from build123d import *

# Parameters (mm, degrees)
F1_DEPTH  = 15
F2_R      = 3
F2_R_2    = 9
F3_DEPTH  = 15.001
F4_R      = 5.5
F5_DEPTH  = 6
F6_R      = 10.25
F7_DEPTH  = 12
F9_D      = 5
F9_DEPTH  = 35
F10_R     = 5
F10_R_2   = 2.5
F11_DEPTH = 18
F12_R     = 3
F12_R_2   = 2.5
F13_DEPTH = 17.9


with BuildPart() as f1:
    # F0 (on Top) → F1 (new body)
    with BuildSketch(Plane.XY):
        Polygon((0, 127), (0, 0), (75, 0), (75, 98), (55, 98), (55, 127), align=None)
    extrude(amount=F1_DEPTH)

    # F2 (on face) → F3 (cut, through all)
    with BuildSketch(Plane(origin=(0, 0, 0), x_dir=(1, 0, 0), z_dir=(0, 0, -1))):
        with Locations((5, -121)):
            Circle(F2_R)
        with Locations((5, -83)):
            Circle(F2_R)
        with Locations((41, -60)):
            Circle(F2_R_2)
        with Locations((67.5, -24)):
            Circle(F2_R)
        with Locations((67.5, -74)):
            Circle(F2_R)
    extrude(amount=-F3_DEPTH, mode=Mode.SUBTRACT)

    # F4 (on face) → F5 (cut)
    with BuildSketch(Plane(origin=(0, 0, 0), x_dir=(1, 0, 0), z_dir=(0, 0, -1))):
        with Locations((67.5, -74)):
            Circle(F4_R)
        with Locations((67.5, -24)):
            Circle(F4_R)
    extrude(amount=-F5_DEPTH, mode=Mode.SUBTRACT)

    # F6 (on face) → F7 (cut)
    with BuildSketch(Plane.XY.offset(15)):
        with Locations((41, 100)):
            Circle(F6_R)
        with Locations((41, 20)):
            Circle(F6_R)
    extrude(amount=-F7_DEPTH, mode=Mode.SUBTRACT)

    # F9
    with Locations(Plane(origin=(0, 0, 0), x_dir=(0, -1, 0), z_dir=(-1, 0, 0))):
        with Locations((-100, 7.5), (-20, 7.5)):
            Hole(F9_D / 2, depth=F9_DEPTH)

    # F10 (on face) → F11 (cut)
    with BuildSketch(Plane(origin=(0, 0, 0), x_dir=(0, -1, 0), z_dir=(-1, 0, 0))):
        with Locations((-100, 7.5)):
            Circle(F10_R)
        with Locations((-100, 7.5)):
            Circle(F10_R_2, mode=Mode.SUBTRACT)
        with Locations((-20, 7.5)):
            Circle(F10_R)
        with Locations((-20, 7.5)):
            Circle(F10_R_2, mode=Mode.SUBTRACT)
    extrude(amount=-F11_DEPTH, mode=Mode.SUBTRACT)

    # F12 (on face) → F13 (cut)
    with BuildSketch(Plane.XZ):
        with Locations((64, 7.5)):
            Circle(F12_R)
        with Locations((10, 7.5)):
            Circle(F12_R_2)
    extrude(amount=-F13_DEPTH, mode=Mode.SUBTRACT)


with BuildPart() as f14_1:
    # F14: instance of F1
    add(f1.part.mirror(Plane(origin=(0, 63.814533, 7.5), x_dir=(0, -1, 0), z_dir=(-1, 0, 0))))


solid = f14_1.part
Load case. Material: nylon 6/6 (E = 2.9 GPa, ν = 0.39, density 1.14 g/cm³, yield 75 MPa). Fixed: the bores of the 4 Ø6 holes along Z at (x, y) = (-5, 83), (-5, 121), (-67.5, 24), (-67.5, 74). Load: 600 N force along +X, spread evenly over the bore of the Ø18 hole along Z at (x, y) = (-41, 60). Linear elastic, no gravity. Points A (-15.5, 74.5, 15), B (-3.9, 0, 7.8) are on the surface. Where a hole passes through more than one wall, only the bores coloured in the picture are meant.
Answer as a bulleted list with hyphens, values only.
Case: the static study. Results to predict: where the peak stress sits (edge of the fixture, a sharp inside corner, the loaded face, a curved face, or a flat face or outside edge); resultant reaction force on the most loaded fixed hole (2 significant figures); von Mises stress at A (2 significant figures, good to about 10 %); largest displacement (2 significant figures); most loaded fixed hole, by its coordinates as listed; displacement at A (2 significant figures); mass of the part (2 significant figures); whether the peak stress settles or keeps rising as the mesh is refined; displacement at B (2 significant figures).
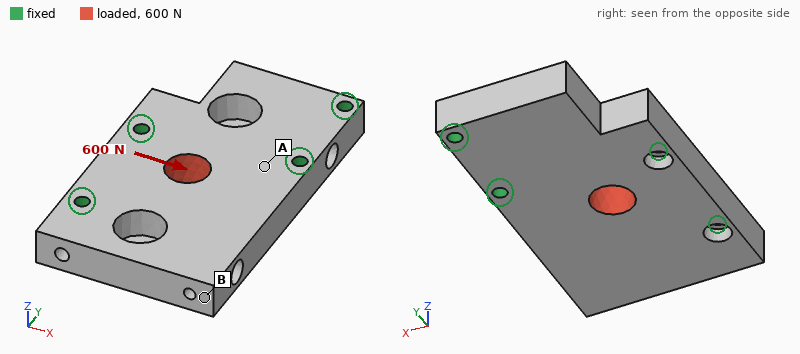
- edge of the fixture
- 250 N
- 0.75 MPa
- 15 µm
- (-67.5, 74)
- 5.5 µm
- 130 g
- keeps rising
- 12 µm
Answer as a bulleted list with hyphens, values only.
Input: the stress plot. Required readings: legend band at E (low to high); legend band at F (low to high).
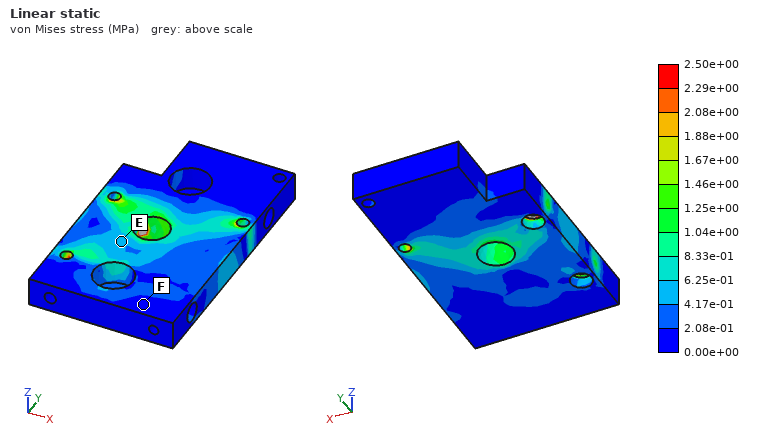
- 4.17e-01 to 6.25e-01 MPa
- 0.00e+00 to 2.08e-01 MPa
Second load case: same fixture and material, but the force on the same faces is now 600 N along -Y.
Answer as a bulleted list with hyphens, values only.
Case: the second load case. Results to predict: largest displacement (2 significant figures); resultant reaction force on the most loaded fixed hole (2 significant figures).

- 13 µm
- 210 N
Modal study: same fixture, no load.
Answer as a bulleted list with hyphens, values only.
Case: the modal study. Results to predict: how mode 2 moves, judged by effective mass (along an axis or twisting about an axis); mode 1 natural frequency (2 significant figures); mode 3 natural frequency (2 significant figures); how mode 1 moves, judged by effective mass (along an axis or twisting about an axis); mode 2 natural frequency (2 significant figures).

- along Z
- 1000 Hz
- 2800 Hz
- along Z
- 2300 Hz
